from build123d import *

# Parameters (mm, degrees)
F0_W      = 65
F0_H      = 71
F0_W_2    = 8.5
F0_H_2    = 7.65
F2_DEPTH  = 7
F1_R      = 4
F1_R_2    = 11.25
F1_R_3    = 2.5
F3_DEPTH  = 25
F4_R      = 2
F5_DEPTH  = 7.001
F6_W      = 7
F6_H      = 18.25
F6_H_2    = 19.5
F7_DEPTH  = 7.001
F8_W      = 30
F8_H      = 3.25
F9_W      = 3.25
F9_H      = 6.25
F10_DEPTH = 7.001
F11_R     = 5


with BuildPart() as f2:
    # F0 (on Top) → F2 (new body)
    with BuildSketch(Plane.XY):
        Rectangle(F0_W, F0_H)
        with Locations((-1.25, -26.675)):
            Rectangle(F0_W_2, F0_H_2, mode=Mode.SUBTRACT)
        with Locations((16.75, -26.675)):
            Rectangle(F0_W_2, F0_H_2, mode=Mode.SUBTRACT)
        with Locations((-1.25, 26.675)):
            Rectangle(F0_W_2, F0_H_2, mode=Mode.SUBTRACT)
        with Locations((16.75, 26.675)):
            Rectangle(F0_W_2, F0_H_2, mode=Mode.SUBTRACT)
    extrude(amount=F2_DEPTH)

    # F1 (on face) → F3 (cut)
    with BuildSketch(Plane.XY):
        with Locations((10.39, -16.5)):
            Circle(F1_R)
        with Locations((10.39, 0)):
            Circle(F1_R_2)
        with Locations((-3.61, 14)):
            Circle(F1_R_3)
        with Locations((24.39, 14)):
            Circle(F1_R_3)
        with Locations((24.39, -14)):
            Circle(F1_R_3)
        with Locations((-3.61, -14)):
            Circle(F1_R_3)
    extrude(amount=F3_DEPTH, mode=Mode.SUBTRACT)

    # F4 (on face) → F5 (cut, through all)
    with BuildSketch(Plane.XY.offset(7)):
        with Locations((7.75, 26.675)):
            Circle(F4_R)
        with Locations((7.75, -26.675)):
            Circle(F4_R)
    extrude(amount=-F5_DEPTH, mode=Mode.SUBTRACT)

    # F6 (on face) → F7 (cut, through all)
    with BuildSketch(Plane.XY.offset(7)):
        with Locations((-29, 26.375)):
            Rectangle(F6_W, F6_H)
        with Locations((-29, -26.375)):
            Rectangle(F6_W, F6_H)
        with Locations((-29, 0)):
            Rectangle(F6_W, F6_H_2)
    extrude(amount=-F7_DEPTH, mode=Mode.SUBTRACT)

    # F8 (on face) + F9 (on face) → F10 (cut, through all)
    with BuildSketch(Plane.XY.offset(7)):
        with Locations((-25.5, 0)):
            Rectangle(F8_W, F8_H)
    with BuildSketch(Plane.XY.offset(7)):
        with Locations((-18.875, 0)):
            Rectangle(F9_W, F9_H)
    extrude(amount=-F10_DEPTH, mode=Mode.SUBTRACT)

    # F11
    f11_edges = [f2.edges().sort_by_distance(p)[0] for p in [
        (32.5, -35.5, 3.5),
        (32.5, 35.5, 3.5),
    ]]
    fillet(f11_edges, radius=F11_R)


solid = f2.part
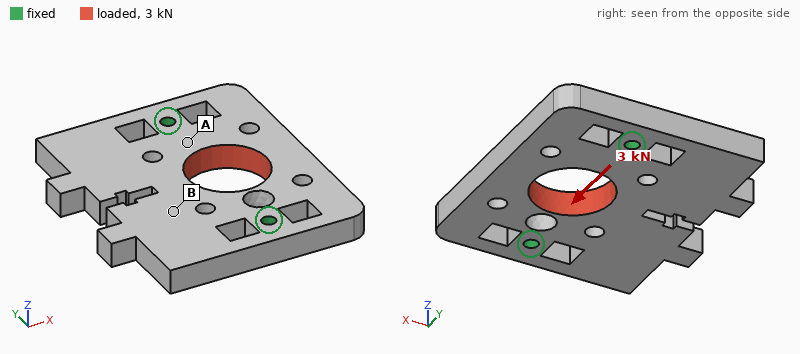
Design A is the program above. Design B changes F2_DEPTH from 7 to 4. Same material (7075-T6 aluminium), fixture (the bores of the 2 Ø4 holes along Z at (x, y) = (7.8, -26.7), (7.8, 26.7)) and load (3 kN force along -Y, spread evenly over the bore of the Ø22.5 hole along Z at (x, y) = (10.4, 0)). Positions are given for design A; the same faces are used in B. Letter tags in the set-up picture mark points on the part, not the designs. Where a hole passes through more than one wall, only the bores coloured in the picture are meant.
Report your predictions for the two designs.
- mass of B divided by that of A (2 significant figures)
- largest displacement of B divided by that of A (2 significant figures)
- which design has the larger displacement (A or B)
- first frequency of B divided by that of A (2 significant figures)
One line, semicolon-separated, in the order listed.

0.57; 1.8; B; 0.63
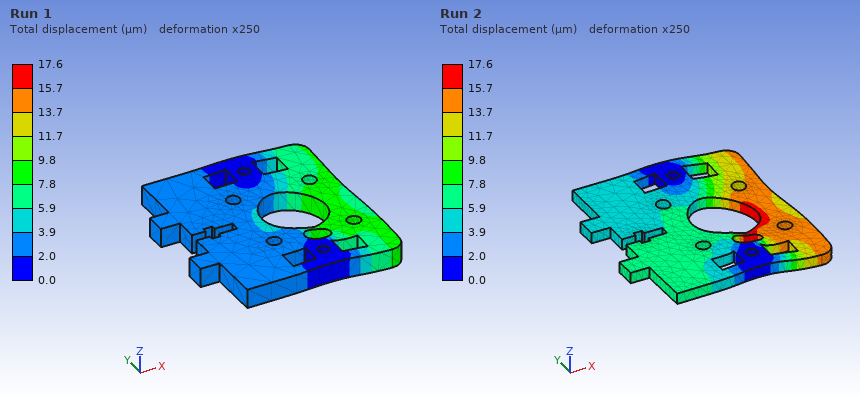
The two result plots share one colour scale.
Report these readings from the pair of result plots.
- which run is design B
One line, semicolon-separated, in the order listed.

Run 2
